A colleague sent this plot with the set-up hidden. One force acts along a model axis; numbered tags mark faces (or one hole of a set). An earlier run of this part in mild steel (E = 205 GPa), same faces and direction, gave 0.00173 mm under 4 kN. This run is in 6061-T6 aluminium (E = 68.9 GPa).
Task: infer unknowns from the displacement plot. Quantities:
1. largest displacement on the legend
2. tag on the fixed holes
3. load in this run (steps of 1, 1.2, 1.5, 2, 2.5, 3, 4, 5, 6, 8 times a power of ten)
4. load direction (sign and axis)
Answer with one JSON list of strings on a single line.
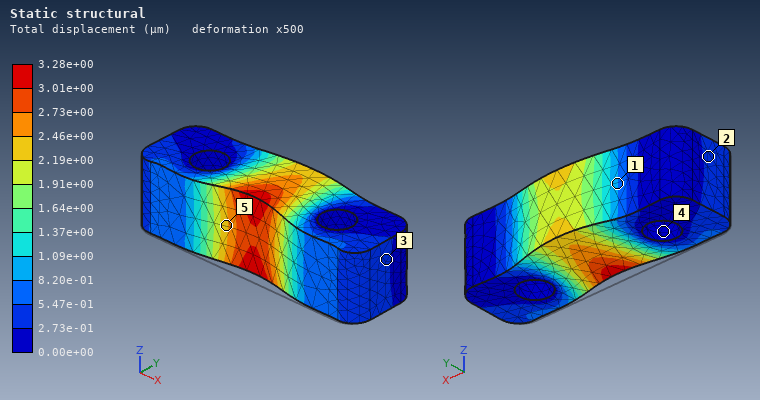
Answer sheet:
["3.28e+00 µm", "4", "2.5 kN", "+Y"]
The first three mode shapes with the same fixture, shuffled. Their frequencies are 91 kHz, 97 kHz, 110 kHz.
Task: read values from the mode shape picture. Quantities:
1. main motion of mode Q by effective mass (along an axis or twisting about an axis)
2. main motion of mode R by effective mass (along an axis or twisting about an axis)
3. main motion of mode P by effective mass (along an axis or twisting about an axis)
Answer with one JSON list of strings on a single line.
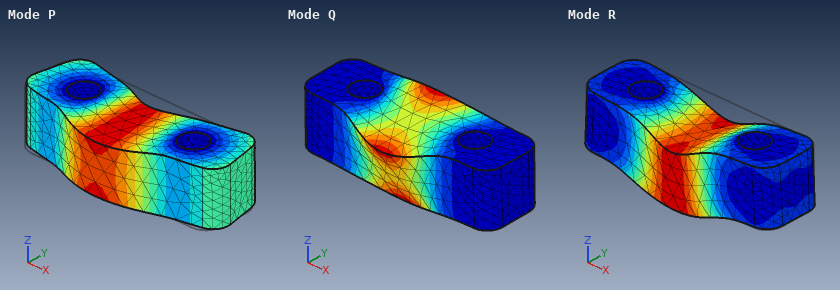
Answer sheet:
["twisting about X", "along Z", "along Y"]
